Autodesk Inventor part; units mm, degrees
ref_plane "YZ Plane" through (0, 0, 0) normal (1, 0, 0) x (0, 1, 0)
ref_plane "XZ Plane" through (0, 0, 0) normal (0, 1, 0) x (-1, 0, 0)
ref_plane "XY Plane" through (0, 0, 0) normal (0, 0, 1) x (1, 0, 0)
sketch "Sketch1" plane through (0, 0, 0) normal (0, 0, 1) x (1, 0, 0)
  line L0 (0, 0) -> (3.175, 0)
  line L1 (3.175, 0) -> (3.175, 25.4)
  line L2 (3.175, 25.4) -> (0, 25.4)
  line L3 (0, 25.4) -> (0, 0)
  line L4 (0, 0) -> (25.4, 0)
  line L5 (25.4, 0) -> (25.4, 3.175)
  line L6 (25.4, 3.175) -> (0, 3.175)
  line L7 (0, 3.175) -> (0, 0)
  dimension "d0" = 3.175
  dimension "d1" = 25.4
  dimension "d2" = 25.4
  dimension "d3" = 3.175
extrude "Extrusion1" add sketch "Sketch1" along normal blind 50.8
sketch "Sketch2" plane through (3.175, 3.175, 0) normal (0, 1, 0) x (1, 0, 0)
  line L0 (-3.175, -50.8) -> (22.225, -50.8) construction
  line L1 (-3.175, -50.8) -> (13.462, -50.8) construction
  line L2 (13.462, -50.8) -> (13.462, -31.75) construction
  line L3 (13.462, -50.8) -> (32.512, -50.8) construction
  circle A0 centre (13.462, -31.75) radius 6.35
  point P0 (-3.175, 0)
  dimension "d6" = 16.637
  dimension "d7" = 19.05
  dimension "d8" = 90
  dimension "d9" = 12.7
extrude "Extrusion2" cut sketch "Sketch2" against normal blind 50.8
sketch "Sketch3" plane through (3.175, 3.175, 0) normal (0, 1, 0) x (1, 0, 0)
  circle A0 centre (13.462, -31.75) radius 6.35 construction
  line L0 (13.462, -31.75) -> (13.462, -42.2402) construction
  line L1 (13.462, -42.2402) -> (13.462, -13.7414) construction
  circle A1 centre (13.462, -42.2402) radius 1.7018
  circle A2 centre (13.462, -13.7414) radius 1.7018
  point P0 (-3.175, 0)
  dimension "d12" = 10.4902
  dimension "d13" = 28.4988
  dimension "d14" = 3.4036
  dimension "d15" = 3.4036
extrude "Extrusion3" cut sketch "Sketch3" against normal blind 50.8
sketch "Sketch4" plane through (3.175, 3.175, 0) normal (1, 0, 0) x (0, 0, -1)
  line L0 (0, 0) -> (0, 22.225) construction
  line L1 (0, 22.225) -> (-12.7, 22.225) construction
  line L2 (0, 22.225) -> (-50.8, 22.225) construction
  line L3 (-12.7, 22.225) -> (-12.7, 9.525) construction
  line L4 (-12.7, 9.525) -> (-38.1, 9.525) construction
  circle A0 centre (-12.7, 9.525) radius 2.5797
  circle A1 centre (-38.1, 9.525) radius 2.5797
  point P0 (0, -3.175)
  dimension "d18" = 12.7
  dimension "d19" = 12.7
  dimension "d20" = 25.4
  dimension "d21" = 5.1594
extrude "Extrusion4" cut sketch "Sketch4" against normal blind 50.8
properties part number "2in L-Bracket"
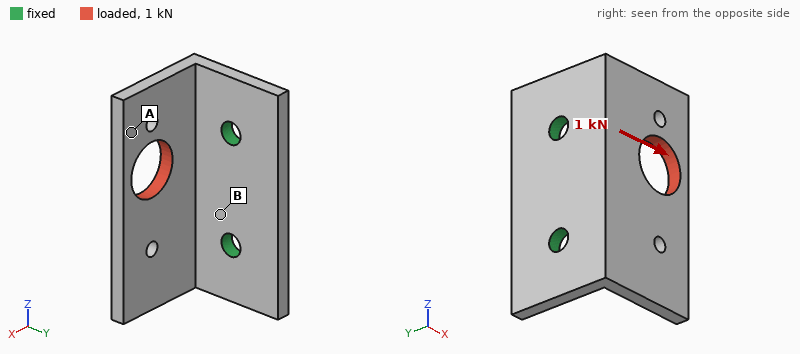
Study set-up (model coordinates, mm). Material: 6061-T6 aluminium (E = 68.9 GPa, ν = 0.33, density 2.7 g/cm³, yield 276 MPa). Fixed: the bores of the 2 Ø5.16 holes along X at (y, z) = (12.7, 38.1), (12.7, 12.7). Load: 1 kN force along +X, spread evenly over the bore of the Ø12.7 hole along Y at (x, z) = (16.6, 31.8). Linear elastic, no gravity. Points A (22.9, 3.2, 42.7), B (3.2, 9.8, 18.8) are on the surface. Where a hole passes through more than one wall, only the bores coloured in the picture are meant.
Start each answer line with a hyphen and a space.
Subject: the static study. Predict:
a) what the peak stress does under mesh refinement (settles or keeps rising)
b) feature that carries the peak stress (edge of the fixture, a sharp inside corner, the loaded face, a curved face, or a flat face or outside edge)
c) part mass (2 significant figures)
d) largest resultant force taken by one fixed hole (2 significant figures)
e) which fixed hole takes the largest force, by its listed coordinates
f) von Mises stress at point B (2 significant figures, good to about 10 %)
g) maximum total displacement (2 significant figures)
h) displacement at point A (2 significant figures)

- keeps rising
- edge of the fixture
- 19 g
- 710 N
- (12.7, 38.1)
- 55 MPa
- 0.19 mm
- 0.16 mm
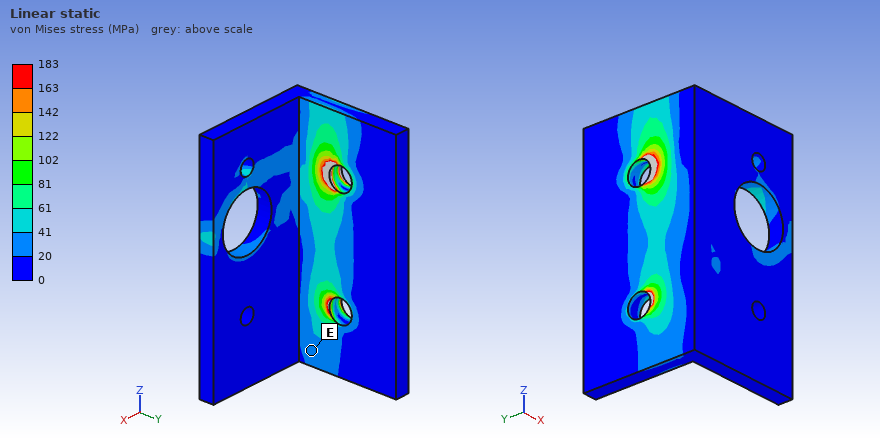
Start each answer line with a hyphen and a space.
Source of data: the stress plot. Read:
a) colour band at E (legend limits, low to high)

- 20 to 41 MPa
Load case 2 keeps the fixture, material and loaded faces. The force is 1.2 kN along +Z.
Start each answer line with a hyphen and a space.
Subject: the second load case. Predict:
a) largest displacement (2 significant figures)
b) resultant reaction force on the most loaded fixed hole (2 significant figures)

- 0.14 mm
- 960 N
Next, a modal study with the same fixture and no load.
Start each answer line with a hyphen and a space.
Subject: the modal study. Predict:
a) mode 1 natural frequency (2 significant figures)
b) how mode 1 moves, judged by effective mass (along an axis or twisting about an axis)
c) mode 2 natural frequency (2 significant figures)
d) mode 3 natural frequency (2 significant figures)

- 2900 Hz
- along Y
- 4500 Hz
- 7600 Hz
